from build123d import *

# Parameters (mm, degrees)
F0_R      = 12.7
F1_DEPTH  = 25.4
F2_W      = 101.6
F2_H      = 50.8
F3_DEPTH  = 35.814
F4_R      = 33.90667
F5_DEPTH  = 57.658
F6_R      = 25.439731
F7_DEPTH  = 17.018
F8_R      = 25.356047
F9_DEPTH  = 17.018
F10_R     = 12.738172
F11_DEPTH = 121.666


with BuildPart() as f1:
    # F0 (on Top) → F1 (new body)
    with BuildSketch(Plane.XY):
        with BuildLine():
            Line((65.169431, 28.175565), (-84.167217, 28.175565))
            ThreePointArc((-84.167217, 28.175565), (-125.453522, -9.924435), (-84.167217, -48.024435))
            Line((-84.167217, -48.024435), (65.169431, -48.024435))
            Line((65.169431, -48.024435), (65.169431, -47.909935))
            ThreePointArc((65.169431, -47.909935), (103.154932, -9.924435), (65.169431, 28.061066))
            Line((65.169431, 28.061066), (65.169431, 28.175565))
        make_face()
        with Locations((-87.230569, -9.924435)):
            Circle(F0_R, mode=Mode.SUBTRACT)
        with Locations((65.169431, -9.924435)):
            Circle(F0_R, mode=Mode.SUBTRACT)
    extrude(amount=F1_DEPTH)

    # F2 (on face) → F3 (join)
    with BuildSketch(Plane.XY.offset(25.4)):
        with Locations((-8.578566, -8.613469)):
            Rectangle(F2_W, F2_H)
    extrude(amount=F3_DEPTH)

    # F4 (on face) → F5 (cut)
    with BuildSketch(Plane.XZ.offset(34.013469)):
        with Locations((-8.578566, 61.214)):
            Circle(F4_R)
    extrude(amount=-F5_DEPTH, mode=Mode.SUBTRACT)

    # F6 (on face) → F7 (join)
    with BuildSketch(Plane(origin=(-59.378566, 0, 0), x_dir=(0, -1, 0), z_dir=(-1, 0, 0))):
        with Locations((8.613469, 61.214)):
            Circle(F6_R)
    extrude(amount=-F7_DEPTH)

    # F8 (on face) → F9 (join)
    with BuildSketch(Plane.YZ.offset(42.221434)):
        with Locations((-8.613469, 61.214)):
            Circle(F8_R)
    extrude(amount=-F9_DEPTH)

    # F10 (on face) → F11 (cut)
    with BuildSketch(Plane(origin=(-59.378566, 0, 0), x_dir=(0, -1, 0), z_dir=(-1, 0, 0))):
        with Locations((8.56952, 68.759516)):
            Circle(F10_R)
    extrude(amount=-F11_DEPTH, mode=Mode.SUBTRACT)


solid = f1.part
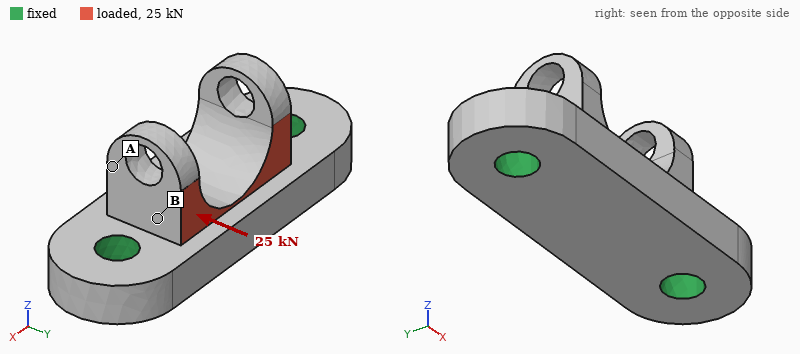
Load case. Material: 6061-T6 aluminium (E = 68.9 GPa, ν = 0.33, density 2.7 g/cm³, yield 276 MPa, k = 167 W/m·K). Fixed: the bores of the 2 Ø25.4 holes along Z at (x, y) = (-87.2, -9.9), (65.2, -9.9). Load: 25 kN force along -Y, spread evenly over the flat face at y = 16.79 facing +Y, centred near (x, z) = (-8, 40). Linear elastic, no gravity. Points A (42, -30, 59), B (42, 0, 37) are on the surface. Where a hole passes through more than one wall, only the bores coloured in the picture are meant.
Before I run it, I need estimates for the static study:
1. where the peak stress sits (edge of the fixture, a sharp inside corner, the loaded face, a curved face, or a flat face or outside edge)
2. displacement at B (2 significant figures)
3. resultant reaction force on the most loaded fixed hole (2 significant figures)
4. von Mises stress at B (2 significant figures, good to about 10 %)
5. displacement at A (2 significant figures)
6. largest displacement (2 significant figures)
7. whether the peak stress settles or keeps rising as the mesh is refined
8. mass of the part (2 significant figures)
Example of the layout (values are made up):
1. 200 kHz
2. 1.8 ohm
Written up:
1. edge of the fixture
2. 36 µm
3. 13 kN
4. 22 MPa
5. 61 µm
6. 91 µm
7. keeps rising
8. 1.3 kg
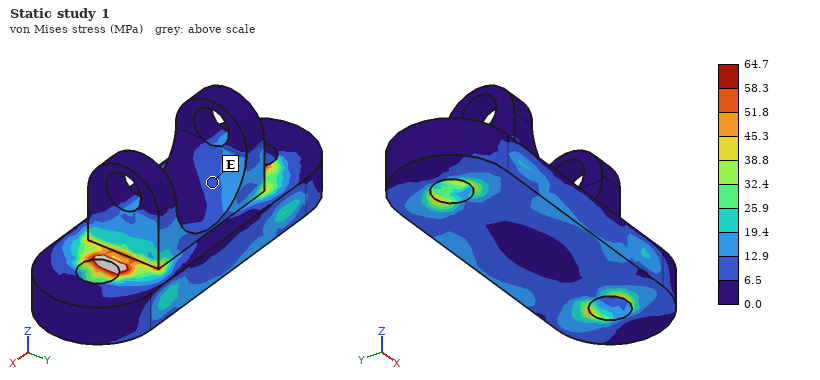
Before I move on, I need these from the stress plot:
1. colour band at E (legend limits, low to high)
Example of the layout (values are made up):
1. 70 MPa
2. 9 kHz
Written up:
1. 6.5 to 12.9 MPa
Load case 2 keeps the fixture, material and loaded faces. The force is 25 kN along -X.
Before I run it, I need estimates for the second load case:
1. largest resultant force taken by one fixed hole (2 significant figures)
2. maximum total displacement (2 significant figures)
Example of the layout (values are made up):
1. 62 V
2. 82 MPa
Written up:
1. 15 kN
2. 59 µm
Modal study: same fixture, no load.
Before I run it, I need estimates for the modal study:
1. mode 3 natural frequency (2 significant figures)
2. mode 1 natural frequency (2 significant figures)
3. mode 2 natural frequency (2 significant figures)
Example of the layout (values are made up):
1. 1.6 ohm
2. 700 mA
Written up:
1. 6500 Hz
2. 4400 Hz
3. 4500 Hz
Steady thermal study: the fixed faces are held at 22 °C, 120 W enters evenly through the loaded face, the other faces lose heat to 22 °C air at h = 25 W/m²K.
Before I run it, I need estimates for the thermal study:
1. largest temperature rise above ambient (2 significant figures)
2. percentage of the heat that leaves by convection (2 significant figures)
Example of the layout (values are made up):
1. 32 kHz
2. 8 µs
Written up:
1. 16 K
2. 5.8 %
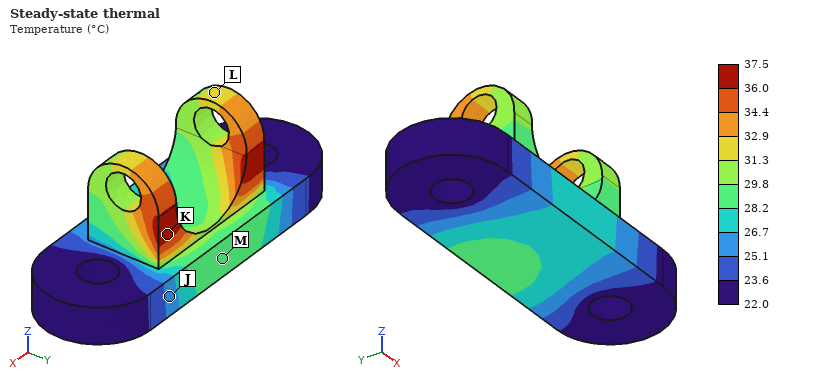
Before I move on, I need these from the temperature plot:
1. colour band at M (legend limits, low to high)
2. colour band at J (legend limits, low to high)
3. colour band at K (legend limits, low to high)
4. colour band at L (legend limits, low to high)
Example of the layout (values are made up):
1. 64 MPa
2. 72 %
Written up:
1. 28.2 to 29.8 °C
2. 25.1 to 26.7 °C
3. 36.0 to 37.5 °C
4. 31.3 to 32.9 °C
